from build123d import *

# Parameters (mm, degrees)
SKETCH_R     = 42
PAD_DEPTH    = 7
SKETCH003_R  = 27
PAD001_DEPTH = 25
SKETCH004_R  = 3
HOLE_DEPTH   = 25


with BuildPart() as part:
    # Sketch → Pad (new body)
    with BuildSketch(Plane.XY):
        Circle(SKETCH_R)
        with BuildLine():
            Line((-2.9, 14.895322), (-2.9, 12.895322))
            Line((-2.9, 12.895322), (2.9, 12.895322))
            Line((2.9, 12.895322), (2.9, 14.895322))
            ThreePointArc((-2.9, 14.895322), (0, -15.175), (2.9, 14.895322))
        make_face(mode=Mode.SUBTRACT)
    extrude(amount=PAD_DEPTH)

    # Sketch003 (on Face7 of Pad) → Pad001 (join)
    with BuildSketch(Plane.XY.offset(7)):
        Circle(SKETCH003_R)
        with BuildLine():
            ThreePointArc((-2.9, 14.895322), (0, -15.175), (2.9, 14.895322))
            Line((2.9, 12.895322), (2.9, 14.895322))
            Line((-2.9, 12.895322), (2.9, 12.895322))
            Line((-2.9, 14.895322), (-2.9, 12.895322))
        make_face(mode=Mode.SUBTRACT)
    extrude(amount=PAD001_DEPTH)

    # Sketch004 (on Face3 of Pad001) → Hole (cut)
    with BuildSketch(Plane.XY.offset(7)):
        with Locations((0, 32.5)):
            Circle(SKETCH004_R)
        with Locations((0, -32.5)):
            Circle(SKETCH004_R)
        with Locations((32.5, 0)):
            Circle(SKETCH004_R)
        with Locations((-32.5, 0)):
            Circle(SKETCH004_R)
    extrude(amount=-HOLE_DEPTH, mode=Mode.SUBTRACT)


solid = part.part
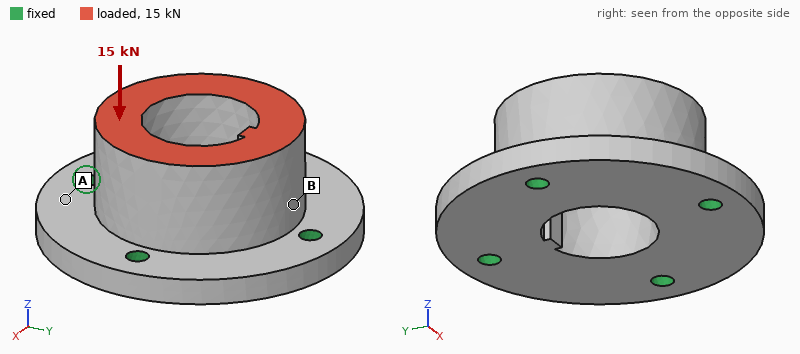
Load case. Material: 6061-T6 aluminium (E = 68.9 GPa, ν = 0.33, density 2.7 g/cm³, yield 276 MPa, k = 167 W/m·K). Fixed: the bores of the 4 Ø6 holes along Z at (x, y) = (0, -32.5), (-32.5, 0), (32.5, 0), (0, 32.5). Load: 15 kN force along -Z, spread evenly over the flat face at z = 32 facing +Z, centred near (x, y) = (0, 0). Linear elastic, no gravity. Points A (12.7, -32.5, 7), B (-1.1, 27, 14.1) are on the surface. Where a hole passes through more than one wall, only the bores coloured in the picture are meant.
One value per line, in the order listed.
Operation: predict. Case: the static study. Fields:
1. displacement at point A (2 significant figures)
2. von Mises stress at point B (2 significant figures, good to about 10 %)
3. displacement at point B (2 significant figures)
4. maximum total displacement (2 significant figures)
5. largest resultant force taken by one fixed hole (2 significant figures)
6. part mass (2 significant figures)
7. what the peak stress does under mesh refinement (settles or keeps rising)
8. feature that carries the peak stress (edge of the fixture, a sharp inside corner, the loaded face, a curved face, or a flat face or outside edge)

7.0 µm
24 MPa
14 µm
18 µm
4.0 kN
200 g
keeps rising
edge of the fixture
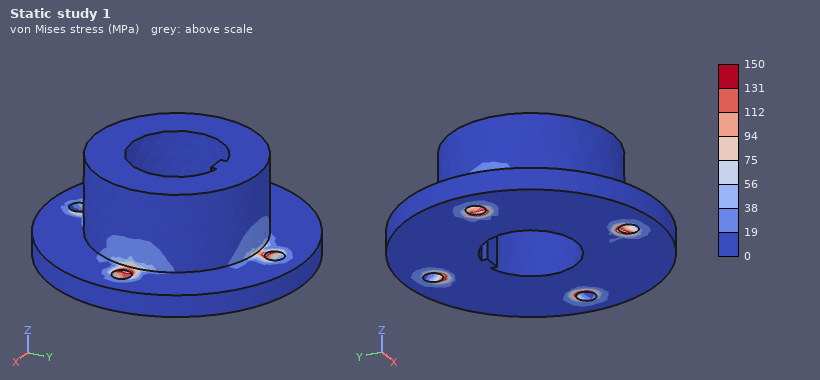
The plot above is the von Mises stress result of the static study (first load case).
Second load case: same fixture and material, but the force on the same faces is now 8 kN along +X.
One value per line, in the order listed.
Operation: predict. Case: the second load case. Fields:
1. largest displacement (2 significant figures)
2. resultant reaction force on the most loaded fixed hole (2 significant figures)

31 µm
4.5 kN
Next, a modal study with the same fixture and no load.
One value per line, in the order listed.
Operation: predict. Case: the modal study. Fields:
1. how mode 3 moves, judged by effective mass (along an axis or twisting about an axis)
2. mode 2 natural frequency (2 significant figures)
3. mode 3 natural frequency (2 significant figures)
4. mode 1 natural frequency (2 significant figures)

along Z
11 kHz
12 kHz
11 kHz
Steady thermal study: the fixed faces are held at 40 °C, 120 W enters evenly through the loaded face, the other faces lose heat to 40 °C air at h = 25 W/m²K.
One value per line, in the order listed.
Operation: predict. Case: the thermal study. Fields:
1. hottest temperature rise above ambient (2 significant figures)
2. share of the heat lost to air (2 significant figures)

21 K
3.3 %
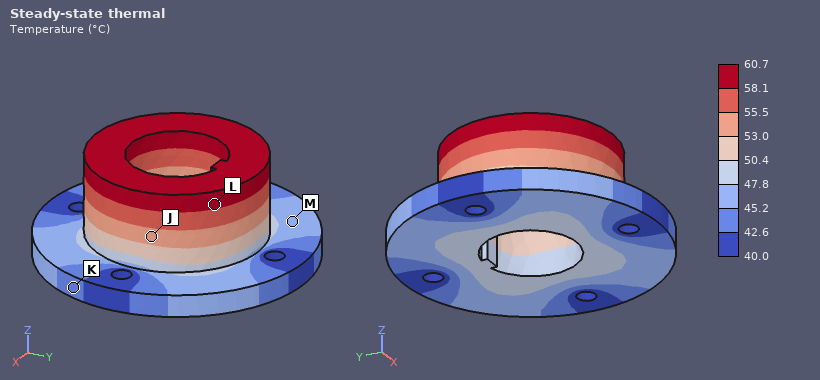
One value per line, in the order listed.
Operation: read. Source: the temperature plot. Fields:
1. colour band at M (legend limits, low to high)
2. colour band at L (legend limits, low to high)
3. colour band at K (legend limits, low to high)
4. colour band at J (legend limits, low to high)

45.2 to 47.8 °C
58.1 to 60.7 °C
42.6 to 45.2 °C
53.0 to 55.5 °C
